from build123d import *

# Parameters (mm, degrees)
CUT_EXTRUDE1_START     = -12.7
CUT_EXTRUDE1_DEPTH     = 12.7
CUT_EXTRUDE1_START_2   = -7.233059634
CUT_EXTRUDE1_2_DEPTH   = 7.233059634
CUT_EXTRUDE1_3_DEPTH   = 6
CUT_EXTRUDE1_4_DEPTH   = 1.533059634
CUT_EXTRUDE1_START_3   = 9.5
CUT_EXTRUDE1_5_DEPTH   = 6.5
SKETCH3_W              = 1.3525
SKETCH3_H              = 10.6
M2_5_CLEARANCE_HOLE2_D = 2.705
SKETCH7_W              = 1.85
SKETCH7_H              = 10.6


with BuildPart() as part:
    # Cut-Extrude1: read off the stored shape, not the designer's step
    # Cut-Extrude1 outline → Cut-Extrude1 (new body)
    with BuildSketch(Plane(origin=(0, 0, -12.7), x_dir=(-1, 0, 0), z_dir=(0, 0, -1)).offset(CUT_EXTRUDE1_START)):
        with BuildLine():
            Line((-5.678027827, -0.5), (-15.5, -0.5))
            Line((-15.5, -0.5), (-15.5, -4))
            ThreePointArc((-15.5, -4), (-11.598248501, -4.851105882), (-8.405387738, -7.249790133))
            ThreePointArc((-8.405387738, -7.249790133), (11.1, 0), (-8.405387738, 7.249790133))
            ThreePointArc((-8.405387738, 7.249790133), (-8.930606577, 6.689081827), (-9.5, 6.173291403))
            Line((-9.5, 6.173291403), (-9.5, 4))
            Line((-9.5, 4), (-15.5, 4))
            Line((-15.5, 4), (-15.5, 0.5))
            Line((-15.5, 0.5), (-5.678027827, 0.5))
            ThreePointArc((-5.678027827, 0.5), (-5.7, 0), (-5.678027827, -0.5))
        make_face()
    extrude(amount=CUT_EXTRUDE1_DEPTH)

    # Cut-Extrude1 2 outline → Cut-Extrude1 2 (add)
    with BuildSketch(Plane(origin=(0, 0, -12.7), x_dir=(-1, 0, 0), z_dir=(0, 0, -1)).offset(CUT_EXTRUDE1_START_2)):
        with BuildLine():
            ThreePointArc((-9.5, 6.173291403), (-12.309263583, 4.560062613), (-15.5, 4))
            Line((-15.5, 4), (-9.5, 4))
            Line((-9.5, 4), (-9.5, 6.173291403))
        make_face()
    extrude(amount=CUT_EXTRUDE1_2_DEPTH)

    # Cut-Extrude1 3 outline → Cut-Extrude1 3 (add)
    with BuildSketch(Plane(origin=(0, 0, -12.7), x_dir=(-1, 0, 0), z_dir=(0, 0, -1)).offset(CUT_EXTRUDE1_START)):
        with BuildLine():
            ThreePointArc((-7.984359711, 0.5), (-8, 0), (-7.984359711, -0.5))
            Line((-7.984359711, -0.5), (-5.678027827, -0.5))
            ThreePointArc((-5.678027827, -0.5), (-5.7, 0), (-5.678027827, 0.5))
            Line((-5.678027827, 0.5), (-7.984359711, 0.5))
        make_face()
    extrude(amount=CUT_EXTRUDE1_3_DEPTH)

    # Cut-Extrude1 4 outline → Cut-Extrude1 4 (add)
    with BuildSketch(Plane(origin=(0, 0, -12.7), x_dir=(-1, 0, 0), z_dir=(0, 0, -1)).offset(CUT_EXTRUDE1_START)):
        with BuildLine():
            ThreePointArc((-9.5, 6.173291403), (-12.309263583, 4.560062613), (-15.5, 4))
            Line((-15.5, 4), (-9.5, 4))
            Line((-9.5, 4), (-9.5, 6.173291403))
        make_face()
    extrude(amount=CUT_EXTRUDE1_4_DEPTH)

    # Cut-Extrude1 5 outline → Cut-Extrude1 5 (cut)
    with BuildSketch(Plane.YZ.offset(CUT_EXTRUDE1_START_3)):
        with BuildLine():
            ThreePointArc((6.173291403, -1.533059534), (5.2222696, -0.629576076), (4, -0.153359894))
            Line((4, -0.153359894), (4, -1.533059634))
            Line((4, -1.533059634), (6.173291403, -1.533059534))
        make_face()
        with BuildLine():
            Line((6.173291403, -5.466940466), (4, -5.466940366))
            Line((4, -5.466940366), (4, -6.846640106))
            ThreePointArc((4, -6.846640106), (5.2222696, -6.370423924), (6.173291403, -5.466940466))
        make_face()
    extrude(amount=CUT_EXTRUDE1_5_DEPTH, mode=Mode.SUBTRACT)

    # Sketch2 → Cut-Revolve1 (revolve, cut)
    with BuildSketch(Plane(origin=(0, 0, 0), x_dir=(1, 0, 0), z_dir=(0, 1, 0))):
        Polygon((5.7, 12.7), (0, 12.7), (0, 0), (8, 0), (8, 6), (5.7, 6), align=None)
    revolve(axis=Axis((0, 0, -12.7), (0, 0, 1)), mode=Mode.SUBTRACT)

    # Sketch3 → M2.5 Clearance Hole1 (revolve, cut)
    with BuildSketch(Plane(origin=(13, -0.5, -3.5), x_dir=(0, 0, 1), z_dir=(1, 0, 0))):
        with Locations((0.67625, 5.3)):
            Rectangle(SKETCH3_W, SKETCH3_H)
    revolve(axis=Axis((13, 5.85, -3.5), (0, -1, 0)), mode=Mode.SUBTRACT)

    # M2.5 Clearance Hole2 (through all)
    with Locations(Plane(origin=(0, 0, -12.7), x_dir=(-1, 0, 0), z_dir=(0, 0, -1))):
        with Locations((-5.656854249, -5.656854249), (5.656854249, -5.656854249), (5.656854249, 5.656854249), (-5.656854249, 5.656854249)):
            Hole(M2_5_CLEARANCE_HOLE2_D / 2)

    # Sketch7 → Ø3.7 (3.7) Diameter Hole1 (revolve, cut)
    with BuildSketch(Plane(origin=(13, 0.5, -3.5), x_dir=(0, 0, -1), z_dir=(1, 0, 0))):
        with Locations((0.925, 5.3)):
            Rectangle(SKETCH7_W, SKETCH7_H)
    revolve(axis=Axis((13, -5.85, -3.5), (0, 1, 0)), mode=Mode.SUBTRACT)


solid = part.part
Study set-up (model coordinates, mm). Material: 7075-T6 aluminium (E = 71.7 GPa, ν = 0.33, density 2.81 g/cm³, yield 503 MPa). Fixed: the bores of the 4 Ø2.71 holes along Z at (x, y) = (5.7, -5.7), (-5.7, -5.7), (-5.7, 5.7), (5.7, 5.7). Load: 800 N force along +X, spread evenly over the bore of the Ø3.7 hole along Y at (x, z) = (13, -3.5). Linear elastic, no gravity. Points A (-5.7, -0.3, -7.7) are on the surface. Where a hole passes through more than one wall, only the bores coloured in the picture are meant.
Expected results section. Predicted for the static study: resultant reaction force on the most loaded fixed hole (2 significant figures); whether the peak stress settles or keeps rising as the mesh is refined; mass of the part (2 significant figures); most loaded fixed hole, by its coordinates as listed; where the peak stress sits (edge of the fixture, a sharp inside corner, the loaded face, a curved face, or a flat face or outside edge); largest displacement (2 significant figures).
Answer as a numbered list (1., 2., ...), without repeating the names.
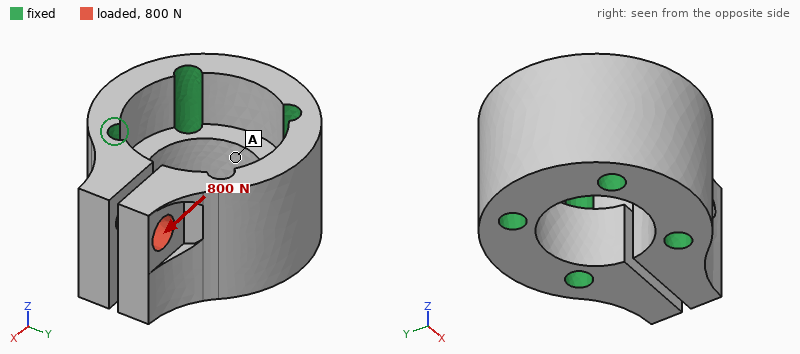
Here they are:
1. 860 N
2. keeps rising
3. 8.9 g
4. (5.7, 5.7)
5. edge of the fixture
6. 27 µm
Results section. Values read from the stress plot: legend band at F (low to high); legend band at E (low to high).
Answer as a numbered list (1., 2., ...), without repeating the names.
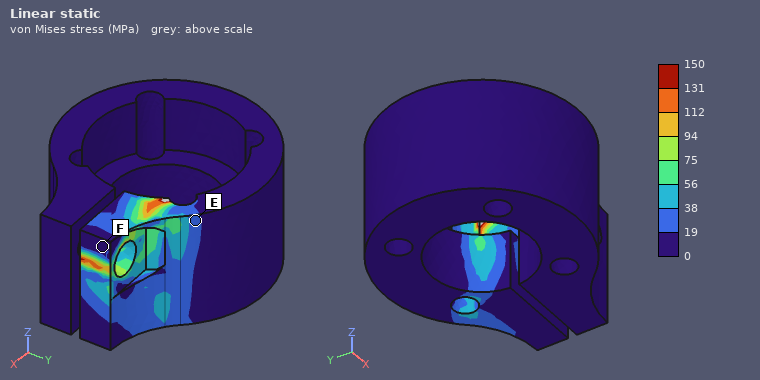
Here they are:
1. 0 to 19 MPa
2. 19 to 38 MPa
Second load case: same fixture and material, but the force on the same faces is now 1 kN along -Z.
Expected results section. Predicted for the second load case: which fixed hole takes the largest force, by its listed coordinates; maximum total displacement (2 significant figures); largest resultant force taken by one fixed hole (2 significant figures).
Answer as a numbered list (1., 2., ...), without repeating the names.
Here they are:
1. (5.7, 5.7)
2. 24 µm
3. 1.0 kN
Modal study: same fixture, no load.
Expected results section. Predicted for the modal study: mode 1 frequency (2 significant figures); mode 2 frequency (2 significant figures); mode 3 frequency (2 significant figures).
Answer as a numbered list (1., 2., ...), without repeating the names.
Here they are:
1. 34 kHz
2. 34 kHz
3. 50 kHz
